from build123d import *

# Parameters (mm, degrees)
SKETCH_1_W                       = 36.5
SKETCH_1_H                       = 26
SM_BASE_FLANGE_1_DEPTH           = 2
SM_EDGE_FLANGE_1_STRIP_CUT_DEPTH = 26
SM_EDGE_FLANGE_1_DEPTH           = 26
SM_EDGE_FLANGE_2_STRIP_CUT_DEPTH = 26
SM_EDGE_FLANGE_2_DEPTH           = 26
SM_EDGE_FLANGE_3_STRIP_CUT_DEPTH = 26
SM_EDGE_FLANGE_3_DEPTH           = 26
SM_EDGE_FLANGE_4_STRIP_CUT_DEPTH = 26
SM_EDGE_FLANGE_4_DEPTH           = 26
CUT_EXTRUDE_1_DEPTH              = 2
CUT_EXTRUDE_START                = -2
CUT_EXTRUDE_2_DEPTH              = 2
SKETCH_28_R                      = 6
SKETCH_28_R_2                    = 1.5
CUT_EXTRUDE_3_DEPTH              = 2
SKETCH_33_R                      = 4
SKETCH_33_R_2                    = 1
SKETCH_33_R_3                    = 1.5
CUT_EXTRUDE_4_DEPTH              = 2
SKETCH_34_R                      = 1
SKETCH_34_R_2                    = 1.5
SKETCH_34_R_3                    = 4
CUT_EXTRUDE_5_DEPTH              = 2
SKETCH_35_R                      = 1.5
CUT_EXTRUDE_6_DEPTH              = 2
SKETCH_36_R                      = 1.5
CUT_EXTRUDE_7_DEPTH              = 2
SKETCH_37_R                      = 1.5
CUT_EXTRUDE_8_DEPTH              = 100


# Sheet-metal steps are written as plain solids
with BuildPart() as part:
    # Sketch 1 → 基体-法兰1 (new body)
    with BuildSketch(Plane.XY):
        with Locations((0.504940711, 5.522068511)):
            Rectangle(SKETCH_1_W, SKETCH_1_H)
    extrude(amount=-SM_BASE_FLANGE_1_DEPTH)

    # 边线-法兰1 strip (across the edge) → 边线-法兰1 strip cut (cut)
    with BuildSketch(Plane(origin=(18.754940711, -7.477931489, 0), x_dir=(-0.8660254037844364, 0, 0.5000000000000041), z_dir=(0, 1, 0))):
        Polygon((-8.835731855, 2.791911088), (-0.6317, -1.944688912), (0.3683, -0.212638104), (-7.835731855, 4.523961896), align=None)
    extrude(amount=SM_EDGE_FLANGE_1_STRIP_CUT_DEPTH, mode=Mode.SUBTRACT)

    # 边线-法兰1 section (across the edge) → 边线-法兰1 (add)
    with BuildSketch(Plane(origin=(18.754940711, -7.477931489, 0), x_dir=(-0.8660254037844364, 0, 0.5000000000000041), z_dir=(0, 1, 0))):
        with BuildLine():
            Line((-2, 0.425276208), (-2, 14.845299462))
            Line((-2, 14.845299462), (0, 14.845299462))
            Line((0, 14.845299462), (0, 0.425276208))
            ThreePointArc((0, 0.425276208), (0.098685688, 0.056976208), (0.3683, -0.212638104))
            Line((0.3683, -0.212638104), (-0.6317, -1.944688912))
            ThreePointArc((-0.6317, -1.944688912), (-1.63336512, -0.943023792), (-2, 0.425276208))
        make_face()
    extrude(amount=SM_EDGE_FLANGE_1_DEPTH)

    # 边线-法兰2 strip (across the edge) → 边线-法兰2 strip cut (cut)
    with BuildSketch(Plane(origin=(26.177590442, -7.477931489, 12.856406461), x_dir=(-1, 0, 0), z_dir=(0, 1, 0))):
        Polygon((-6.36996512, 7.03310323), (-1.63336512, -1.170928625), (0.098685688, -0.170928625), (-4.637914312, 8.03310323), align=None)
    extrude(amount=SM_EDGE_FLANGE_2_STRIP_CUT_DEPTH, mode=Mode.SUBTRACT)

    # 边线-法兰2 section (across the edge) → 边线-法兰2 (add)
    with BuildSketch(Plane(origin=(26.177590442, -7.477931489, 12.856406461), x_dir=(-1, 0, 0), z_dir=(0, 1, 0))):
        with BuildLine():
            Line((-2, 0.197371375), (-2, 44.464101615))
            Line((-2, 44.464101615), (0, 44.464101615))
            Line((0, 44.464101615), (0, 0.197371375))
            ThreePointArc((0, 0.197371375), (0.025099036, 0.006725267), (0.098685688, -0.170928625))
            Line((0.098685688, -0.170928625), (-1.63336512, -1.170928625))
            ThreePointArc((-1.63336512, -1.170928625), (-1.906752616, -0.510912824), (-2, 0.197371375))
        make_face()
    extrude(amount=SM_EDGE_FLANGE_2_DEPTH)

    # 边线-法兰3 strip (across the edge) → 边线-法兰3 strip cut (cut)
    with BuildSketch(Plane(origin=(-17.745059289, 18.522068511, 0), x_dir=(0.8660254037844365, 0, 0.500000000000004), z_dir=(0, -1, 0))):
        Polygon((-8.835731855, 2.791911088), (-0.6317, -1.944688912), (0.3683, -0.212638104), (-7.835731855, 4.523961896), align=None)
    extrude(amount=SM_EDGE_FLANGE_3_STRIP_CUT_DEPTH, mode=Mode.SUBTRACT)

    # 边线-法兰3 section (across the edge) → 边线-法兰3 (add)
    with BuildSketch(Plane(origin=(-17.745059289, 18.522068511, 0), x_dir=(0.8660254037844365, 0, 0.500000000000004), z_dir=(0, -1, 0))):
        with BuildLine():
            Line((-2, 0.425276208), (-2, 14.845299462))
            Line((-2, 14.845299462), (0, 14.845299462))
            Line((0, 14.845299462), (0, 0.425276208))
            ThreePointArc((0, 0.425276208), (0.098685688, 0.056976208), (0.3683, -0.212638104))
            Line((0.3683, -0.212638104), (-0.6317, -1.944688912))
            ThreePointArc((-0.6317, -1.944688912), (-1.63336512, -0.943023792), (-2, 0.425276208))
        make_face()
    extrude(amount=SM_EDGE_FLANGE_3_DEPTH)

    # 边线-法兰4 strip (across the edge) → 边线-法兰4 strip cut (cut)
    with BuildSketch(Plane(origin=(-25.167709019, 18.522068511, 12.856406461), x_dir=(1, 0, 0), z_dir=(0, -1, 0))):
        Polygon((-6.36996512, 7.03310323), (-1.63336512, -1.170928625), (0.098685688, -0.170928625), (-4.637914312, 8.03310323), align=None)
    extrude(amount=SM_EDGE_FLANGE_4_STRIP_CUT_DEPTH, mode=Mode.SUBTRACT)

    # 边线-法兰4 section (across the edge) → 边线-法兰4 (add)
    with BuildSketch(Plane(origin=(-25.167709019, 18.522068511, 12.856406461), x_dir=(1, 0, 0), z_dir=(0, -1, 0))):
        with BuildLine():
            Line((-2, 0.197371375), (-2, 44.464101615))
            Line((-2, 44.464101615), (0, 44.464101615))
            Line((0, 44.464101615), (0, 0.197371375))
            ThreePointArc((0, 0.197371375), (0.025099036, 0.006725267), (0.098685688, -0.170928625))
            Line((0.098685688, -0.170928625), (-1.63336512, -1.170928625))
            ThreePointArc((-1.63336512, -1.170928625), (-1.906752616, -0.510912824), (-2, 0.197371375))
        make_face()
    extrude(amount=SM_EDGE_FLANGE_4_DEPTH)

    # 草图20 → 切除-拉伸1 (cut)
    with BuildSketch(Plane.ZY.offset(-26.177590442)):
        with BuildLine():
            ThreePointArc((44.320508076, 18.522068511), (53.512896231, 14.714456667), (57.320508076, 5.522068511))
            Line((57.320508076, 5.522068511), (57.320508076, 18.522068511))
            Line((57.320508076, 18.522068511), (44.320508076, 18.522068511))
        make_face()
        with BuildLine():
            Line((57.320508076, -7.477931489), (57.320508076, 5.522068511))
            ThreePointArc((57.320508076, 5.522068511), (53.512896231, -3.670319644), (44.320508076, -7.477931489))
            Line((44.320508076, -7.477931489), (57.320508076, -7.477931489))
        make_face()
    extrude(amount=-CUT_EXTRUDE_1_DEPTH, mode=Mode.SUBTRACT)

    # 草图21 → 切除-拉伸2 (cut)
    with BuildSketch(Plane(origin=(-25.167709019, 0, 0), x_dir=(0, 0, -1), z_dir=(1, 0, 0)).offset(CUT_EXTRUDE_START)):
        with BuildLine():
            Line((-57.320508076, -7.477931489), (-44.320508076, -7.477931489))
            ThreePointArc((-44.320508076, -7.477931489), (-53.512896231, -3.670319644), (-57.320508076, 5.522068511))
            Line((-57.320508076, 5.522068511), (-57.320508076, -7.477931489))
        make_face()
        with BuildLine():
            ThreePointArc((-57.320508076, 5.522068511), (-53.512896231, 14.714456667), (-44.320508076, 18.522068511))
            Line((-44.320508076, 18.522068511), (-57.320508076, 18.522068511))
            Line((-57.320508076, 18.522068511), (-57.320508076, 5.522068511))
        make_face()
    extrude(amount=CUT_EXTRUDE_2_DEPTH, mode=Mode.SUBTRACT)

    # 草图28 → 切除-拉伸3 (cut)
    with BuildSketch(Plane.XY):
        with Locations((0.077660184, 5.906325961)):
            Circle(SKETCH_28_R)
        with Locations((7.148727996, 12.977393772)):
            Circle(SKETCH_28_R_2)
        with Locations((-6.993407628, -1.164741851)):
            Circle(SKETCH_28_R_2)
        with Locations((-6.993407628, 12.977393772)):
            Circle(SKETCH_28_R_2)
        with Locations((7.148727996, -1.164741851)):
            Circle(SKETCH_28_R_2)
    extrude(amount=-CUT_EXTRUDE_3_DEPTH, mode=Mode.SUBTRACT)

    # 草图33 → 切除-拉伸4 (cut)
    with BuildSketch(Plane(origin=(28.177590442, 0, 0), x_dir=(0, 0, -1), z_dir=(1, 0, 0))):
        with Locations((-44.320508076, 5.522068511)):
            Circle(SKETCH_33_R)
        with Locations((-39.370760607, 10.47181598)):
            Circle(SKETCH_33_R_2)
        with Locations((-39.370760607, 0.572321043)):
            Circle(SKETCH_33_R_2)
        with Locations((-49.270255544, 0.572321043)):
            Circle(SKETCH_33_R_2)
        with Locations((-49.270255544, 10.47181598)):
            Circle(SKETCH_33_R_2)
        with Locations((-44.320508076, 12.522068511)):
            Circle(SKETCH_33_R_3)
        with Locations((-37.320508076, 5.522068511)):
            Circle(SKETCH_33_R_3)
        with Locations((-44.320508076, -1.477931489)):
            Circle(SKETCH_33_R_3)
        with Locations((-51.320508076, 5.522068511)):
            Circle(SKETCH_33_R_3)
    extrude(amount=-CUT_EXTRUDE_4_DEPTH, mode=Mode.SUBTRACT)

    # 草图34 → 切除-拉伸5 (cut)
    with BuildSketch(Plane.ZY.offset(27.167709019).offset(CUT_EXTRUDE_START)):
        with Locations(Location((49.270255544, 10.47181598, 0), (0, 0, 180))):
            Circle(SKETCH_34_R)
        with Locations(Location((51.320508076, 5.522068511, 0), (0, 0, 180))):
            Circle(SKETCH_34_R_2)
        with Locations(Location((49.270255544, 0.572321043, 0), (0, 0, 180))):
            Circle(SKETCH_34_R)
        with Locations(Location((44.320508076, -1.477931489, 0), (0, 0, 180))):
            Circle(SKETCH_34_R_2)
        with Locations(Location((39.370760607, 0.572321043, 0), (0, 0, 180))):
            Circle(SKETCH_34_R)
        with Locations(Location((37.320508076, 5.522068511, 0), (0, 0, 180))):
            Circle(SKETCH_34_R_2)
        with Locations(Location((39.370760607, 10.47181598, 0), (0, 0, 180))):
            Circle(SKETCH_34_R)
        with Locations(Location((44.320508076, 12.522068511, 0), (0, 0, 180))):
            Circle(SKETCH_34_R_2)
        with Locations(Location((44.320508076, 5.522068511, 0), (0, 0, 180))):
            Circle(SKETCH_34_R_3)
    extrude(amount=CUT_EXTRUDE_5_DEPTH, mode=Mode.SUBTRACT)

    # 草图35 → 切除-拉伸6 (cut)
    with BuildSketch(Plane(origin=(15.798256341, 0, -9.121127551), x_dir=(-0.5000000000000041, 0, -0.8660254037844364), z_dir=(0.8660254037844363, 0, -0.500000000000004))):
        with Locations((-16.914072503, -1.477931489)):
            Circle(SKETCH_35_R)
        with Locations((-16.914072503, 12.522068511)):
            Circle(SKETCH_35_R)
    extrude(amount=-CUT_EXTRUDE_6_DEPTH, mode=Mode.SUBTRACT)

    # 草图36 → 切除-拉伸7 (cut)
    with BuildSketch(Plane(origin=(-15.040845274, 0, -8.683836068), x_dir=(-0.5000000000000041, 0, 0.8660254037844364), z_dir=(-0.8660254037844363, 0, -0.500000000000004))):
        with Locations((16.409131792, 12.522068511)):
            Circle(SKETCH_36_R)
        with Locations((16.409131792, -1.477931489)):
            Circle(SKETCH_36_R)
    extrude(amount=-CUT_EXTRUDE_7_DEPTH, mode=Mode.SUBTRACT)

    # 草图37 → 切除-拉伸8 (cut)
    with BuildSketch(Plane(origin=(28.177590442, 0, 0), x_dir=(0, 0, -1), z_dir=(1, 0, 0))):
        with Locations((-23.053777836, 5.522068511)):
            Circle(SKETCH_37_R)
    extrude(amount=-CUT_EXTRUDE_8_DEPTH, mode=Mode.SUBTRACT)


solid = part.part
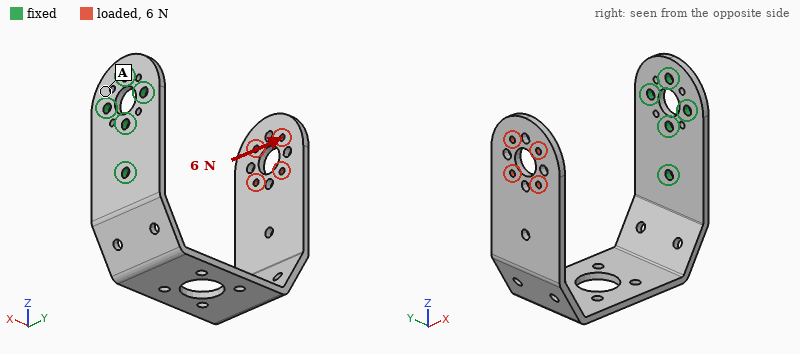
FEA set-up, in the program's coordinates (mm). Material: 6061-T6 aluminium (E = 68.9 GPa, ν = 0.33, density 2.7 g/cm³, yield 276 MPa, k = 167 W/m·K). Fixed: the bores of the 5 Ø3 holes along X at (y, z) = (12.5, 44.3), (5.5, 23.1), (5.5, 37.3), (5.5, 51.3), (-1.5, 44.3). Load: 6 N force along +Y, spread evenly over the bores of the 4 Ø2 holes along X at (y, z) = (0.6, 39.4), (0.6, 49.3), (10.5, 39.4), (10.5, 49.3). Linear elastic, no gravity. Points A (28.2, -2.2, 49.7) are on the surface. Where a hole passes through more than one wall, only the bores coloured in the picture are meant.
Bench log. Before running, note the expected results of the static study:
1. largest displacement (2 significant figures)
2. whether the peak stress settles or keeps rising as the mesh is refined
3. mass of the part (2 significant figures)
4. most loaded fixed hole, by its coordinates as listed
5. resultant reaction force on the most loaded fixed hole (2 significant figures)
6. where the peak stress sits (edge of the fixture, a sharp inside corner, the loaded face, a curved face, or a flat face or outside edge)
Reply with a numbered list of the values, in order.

1. 0.80 mm
2. keeps rising
3. 19 g
4. (5.5, 37.3)
5. 3.7 N
6. edge of the fixture
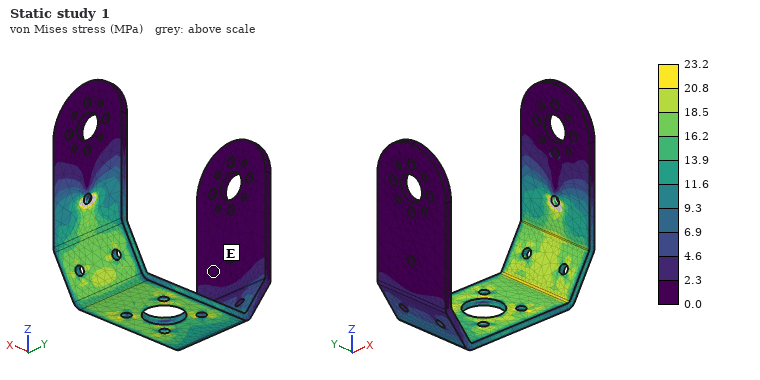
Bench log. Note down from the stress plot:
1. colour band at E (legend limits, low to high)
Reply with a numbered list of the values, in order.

1. 0.0 to 2.3 MPa
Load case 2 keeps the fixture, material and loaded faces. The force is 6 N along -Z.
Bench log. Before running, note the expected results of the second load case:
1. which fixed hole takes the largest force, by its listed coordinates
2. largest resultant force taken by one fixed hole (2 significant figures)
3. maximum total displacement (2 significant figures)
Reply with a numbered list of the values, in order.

1. (5.5, 23.1)
2. 11 N
3. 0.91 mm
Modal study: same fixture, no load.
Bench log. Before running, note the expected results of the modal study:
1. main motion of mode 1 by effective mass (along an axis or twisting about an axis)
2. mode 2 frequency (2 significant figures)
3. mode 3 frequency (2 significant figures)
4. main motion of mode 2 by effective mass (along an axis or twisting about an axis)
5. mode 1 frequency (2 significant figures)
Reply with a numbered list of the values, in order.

1. along Z
2. 220 Hz
3. 420 Hz
4. along Y
5. 150 Hz
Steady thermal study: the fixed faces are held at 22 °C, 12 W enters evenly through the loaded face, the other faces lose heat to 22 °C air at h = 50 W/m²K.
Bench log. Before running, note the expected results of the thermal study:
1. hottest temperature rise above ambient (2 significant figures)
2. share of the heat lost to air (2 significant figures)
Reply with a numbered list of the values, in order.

1. 71 K
2. 81 %
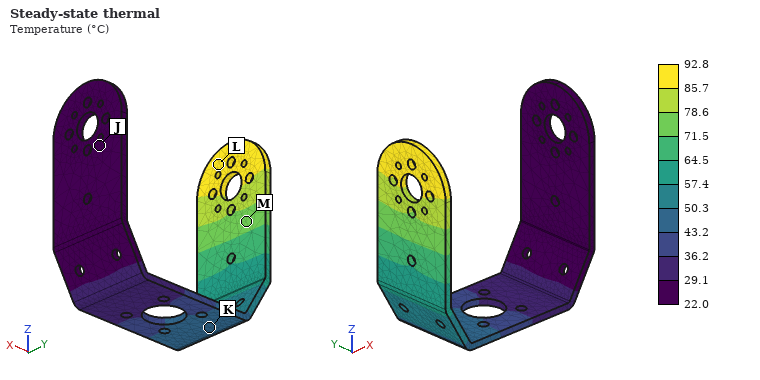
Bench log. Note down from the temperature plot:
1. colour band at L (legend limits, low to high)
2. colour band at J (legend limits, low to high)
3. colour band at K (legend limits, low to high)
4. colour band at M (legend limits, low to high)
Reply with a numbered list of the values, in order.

1. 85.7 to 92.8 °C
2. 22.0 to 29.1 °C
3. 43.2 to 50.3 °C
4. 71.5 to 78.6 °C
